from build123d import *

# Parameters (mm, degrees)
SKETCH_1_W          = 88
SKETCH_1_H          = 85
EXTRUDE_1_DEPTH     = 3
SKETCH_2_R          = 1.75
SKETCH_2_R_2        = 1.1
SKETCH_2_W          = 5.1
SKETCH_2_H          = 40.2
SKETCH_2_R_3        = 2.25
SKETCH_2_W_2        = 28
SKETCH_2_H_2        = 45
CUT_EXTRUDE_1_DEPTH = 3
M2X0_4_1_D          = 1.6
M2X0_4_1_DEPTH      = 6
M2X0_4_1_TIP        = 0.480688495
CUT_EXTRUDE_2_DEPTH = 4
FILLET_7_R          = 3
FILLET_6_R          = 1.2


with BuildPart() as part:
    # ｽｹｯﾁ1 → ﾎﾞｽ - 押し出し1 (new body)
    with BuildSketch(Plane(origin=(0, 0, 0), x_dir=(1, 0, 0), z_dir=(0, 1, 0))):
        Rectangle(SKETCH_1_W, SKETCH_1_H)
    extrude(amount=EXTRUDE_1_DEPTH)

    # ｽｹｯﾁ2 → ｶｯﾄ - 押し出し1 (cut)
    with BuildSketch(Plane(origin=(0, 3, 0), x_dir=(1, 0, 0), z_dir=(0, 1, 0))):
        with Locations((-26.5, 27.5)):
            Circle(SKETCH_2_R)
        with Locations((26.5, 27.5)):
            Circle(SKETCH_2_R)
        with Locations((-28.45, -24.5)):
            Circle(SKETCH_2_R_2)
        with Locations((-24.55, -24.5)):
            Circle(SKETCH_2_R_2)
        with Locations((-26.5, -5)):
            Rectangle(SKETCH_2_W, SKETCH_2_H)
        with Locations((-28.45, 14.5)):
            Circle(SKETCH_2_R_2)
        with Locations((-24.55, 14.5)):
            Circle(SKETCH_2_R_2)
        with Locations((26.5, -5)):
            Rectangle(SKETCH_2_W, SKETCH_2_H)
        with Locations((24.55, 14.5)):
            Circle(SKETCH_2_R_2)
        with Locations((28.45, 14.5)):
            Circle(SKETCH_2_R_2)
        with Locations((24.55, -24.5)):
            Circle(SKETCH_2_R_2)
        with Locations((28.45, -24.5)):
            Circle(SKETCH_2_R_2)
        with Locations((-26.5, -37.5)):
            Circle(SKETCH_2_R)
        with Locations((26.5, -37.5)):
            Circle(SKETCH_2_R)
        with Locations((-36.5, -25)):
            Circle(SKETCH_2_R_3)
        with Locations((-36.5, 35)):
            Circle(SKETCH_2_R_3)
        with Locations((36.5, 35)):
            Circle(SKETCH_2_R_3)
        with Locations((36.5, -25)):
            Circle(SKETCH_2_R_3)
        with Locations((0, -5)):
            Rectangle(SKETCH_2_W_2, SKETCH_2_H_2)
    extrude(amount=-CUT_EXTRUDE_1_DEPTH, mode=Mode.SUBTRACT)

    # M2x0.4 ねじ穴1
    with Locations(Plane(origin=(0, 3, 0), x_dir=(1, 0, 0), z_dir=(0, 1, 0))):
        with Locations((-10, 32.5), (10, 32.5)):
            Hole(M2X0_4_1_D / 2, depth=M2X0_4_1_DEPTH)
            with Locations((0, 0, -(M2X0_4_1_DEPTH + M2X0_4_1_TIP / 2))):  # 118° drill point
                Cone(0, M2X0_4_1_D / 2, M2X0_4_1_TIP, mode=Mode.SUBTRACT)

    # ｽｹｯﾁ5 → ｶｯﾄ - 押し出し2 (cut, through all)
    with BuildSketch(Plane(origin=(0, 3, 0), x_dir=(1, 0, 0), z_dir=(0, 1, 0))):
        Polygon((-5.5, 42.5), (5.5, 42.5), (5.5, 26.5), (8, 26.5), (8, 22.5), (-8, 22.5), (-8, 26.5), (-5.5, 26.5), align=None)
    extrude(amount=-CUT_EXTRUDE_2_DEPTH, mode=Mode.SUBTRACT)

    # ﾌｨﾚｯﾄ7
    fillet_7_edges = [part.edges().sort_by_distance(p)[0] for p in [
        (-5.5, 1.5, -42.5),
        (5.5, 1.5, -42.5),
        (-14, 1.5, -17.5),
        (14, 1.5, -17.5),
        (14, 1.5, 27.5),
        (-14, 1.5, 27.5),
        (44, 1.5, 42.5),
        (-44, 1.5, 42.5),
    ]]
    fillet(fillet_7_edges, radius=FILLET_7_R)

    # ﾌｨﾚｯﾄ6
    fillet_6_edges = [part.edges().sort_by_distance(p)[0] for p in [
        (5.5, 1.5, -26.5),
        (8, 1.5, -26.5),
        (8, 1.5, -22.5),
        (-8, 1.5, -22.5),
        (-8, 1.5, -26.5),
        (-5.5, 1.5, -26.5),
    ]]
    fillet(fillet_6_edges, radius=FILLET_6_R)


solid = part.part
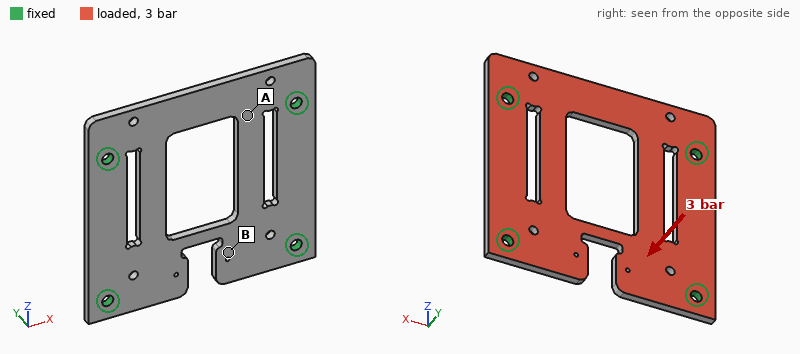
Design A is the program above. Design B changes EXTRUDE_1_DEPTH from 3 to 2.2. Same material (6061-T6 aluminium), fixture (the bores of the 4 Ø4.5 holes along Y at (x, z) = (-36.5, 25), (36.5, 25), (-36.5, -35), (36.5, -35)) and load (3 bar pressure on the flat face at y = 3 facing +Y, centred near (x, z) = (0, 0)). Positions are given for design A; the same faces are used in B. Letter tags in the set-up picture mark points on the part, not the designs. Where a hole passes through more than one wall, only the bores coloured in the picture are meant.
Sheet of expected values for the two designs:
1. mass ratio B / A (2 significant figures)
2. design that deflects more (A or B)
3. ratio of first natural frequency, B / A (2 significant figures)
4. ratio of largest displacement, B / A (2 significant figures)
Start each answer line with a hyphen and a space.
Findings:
- 0.73
- B
- 0.75
- 2.4
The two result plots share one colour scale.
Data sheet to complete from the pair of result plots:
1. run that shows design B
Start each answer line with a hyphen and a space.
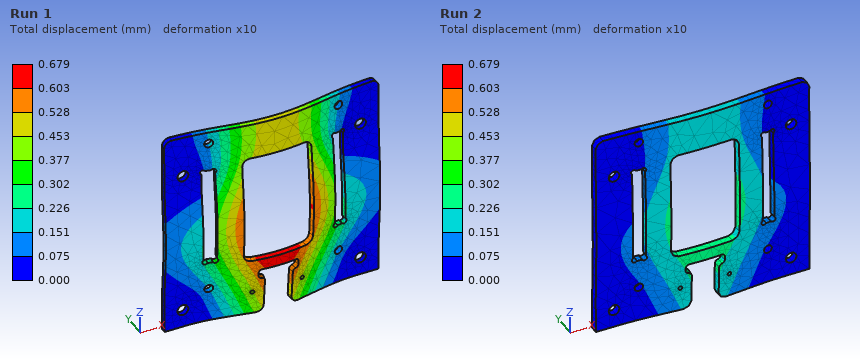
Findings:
- Run 1
